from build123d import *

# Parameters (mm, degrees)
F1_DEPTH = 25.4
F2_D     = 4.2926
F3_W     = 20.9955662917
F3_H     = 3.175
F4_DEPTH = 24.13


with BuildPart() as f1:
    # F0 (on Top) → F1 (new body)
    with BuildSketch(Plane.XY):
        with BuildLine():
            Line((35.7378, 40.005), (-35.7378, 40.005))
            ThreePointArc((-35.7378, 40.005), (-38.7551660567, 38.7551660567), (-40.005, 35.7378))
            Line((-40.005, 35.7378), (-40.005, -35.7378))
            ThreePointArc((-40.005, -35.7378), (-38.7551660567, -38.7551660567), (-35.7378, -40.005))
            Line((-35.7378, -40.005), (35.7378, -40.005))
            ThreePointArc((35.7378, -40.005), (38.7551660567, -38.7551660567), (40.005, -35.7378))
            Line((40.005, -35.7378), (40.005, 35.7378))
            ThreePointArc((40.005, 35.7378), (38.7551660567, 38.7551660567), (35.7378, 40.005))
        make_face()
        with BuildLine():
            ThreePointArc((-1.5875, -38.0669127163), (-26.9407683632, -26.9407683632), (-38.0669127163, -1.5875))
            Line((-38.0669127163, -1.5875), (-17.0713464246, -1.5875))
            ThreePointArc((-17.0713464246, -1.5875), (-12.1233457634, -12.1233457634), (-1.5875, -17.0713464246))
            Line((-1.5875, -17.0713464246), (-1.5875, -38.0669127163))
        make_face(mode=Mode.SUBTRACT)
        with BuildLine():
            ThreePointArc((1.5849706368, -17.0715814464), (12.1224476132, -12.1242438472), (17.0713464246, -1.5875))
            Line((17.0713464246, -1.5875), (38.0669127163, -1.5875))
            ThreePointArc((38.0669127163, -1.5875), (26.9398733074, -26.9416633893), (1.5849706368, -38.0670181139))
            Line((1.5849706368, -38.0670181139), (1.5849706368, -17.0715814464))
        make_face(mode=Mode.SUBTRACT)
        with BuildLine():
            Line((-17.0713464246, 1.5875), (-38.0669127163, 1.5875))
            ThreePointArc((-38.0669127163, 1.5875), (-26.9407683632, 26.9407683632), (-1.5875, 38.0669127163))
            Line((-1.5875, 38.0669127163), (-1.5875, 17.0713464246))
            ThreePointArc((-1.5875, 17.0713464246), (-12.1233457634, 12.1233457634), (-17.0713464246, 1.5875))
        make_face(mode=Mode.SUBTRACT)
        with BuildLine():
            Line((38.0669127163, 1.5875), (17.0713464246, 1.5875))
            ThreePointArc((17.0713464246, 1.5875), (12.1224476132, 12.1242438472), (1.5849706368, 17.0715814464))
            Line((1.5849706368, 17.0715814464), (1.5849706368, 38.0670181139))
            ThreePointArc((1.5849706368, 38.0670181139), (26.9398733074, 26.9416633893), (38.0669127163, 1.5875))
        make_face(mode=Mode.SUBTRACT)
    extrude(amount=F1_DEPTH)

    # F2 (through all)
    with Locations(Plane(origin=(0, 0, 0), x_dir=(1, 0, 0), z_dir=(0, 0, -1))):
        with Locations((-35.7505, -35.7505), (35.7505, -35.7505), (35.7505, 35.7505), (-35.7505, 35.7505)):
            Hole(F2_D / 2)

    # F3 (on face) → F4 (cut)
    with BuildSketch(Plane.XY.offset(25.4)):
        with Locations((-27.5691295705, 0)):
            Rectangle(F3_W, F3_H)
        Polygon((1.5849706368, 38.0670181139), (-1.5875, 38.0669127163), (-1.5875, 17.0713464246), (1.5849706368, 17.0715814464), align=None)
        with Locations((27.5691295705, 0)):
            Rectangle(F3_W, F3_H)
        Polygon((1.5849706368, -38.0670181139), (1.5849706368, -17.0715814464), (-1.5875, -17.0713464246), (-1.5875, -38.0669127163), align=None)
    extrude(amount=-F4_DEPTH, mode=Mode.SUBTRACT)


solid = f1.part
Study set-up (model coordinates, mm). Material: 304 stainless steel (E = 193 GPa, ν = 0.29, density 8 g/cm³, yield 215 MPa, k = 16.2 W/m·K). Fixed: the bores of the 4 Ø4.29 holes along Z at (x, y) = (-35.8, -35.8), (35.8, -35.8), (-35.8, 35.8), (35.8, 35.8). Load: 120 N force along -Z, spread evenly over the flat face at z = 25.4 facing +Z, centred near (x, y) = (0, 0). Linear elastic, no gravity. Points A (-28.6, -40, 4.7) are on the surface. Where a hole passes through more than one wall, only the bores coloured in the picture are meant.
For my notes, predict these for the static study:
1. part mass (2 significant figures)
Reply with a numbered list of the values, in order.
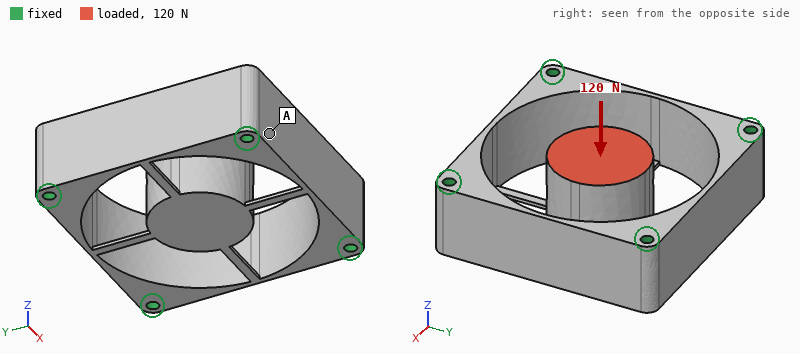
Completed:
1. 550 g
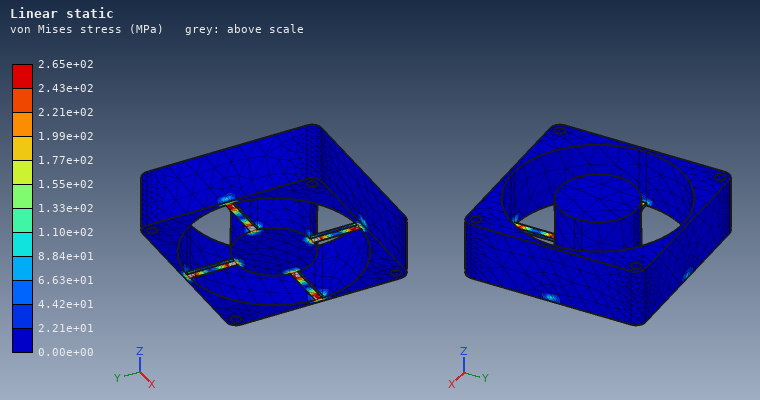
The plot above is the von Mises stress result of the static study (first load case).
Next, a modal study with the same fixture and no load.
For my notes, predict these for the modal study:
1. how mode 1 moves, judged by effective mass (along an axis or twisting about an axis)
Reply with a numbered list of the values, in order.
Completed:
1. along Z
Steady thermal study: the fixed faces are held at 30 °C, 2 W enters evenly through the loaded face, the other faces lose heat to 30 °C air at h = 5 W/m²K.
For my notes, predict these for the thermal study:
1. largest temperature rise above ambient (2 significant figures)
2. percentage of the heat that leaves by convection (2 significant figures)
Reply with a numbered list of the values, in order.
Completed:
1. 68 K
2. 69 %
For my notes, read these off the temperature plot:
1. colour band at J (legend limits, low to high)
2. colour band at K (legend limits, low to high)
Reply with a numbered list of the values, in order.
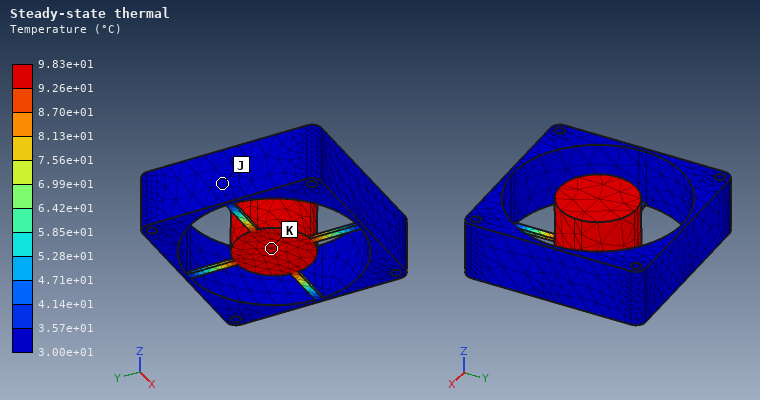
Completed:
1. 3.00e+01 to 3.57e+01 °C
2. 9.26e+01 to 9.83e+01 °C
